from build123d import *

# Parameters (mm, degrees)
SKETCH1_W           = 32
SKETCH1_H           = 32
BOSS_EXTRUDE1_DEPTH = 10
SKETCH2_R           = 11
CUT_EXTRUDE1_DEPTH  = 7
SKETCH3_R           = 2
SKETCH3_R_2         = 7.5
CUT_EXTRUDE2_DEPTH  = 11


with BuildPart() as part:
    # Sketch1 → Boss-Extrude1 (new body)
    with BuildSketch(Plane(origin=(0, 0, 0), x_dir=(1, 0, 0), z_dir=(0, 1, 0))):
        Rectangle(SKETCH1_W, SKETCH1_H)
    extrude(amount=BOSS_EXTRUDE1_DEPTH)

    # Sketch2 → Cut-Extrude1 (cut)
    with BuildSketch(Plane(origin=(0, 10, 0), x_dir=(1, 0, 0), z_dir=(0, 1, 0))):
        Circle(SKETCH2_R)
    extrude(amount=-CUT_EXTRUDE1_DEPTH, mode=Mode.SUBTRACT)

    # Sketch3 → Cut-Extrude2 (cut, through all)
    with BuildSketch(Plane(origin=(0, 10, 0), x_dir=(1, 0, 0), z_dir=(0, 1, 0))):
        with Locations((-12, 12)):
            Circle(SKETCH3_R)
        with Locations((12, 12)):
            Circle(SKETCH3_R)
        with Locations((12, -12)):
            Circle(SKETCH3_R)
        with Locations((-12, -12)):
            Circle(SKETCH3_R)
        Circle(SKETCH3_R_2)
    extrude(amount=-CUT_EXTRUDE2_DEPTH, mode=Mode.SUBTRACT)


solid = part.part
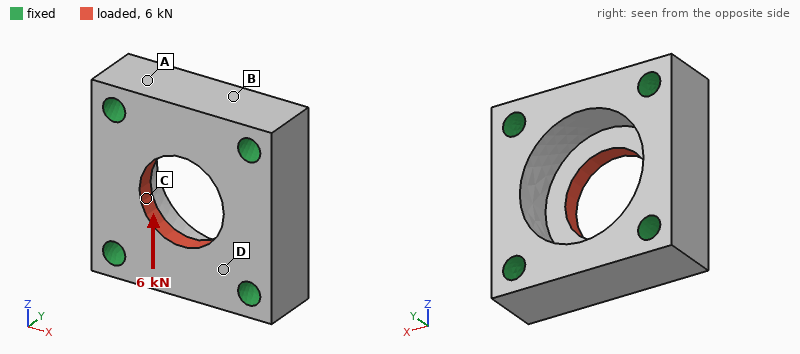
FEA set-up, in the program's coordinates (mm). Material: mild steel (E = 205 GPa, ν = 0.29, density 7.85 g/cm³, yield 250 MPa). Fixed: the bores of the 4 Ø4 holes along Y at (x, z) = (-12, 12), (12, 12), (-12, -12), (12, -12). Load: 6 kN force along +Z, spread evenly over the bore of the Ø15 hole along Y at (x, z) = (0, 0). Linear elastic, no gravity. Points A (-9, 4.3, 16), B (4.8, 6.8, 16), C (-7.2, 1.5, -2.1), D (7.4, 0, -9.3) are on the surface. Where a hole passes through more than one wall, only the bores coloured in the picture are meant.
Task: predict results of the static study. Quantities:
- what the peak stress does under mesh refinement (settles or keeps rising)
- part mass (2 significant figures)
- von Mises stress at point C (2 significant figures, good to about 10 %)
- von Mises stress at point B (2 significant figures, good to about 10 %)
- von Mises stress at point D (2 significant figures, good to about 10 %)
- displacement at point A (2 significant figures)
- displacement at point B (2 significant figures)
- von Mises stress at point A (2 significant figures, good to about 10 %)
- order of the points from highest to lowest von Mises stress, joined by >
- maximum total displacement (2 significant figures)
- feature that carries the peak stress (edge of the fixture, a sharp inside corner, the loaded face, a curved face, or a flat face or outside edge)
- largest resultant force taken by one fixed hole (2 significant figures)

keeps rising
51 g
74 MPa
15 MPa
53 MPa
0.66 µm
1.00 µm
24 MPa
C > D > A > B
4.1 µm
edge of the fixture
1.6 kN
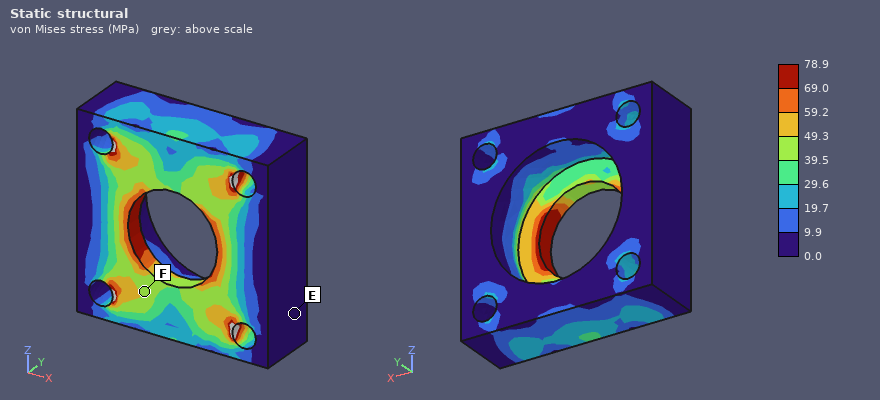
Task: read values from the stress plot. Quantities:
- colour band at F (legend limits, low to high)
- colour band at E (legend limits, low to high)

39.5 to 49.3 MPa
0.0 to 9.9 MPa
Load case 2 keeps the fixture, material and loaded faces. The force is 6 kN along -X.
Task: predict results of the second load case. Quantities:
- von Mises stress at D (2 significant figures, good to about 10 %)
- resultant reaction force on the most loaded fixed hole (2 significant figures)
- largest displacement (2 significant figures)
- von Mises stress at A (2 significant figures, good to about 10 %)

43 MPa
1.6 kN
4.2 µm
6.7 MPa
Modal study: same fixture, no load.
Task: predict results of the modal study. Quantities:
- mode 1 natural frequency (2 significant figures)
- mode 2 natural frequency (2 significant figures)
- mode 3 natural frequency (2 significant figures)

46 kHz
58 kHz
59 kHz
